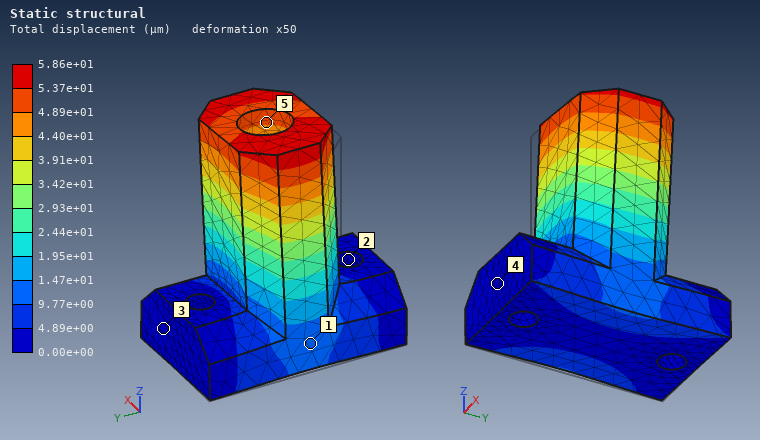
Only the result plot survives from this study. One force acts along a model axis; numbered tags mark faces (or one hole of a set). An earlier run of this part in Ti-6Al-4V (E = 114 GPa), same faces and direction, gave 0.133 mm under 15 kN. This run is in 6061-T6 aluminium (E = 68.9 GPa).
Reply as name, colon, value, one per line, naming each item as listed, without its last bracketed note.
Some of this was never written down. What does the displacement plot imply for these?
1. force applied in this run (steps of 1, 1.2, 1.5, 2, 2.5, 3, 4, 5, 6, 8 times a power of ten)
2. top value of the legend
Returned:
force applied in this run: 4 kN
top value of the legend: 5.86e+01 µm
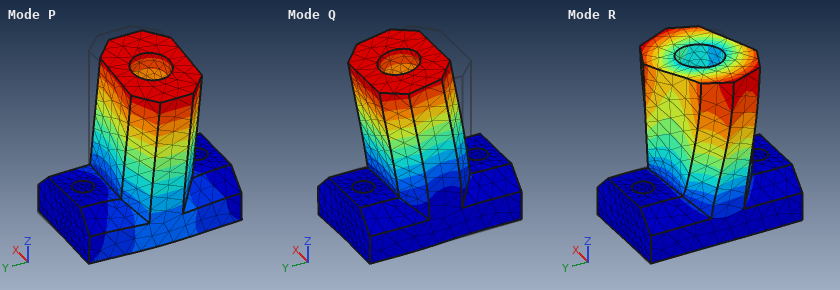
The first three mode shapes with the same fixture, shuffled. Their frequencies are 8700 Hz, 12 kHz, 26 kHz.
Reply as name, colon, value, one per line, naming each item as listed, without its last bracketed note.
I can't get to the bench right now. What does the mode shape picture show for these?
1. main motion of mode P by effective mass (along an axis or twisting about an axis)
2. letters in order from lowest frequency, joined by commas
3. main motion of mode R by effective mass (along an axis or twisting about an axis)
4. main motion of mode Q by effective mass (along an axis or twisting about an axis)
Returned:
main motion of mode P by effective mass: along X
letters in order from lowest frequency, joined by commas: P, Q, R
main motion of mode R by effective mass: twisting about Z
main motion of mode Q by effective mass: along Y
